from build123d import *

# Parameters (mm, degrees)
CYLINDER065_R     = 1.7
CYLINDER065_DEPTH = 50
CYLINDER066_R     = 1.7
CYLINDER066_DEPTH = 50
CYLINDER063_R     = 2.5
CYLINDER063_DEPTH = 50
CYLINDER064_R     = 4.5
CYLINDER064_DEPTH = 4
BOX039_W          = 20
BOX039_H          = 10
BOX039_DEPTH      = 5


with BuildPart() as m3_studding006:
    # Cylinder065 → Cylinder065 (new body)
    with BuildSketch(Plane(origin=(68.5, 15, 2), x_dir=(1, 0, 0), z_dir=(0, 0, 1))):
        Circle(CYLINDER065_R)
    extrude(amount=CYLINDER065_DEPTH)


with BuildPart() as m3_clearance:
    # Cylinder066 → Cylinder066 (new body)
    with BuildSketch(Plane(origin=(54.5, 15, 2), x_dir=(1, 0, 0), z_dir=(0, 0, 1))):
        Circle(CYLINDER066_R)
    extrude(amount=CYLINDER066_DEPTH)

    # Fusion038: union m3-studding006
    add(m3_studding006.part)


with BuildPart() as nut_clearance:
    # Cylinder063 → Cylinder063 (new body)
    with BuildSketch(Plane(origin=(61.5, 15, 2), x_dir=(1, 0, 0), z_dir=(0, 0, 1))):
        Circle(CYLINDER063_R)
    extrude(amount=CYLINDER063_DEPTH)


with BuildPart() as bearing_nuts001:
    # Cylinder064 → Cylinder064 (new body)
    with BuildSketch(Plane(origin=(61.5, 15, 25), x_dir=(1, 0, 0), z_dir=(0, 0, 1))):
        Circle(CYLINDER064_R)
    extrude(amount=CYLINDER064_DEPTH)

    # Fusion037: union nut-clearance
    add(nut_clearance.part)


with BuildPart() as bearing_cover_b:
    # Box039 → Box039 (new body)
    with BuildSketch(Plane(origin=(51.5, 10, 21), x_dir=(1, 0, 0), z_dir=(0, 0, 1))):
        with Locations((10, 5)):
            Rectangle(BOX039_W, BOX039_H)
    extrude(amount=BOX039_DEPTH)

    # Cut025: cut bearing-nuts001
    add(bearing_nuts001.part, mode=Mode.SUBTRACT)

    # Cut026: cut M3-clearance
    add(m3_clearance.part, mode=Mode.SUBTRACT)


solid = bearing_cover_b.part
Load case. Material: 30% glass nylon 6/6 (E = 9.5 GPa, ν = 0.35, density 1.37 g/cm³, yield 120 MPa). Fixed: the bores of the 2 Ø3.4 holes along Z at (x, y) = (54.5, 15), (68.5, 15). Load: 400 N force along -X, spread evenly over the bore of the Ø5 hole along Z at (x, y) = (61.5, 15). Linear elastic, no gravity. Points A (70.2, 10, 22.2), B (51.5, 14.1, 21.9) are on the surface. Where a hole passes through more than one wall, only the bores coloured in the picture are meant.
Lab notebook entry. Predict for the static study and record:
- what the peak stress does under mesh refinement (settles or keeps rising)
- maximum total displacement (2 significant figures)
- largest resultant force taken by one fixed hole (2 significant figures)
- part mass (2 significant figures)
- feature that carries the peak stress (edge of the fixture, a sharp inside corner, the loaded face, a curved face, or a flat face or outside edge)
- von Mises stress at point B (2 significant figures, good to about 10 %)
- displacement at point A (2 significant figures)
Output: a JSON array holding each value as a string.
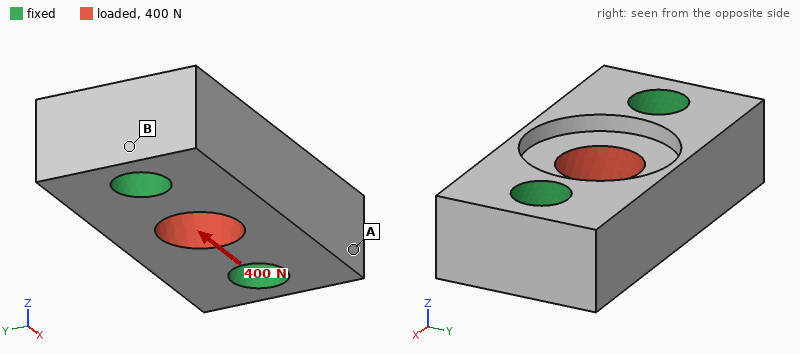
["keeps rising", "4.5 µm", "200 N", "1.1 g", "edge of the fixture", "2.7 MPa", "1.8 µm"]
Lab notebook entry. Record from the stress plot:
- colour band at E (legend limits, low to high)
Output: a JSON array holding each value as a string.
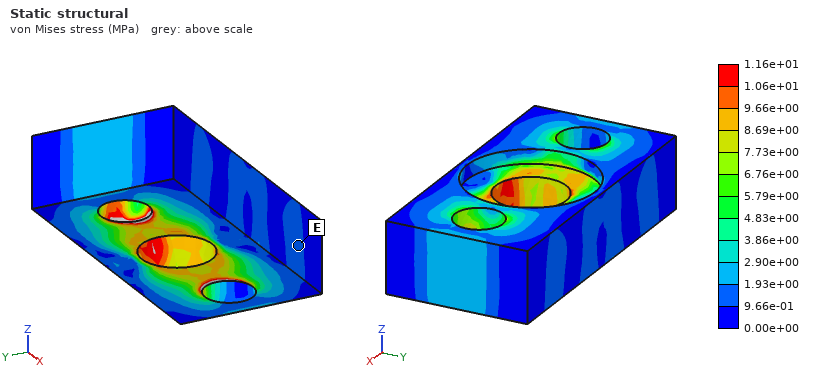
["9.66e-01 to 1.93e+00 MPa"]
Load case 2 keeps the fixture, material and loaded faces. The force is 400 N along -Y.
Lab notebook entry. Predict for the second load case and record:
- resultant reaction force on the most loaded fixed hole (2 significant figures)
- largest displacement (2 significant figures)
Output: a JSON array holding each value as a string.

["200 N", "12 µm"]
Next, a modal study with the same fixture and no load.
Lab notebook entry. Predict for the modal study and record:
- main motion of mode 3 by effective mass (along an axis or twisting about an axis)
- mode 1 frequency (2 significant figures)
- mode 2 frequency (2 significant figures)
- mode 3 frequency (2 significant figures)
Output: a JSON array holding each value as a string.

["along Y", "47 kHz", "48 kHz", "59 kHz"]
